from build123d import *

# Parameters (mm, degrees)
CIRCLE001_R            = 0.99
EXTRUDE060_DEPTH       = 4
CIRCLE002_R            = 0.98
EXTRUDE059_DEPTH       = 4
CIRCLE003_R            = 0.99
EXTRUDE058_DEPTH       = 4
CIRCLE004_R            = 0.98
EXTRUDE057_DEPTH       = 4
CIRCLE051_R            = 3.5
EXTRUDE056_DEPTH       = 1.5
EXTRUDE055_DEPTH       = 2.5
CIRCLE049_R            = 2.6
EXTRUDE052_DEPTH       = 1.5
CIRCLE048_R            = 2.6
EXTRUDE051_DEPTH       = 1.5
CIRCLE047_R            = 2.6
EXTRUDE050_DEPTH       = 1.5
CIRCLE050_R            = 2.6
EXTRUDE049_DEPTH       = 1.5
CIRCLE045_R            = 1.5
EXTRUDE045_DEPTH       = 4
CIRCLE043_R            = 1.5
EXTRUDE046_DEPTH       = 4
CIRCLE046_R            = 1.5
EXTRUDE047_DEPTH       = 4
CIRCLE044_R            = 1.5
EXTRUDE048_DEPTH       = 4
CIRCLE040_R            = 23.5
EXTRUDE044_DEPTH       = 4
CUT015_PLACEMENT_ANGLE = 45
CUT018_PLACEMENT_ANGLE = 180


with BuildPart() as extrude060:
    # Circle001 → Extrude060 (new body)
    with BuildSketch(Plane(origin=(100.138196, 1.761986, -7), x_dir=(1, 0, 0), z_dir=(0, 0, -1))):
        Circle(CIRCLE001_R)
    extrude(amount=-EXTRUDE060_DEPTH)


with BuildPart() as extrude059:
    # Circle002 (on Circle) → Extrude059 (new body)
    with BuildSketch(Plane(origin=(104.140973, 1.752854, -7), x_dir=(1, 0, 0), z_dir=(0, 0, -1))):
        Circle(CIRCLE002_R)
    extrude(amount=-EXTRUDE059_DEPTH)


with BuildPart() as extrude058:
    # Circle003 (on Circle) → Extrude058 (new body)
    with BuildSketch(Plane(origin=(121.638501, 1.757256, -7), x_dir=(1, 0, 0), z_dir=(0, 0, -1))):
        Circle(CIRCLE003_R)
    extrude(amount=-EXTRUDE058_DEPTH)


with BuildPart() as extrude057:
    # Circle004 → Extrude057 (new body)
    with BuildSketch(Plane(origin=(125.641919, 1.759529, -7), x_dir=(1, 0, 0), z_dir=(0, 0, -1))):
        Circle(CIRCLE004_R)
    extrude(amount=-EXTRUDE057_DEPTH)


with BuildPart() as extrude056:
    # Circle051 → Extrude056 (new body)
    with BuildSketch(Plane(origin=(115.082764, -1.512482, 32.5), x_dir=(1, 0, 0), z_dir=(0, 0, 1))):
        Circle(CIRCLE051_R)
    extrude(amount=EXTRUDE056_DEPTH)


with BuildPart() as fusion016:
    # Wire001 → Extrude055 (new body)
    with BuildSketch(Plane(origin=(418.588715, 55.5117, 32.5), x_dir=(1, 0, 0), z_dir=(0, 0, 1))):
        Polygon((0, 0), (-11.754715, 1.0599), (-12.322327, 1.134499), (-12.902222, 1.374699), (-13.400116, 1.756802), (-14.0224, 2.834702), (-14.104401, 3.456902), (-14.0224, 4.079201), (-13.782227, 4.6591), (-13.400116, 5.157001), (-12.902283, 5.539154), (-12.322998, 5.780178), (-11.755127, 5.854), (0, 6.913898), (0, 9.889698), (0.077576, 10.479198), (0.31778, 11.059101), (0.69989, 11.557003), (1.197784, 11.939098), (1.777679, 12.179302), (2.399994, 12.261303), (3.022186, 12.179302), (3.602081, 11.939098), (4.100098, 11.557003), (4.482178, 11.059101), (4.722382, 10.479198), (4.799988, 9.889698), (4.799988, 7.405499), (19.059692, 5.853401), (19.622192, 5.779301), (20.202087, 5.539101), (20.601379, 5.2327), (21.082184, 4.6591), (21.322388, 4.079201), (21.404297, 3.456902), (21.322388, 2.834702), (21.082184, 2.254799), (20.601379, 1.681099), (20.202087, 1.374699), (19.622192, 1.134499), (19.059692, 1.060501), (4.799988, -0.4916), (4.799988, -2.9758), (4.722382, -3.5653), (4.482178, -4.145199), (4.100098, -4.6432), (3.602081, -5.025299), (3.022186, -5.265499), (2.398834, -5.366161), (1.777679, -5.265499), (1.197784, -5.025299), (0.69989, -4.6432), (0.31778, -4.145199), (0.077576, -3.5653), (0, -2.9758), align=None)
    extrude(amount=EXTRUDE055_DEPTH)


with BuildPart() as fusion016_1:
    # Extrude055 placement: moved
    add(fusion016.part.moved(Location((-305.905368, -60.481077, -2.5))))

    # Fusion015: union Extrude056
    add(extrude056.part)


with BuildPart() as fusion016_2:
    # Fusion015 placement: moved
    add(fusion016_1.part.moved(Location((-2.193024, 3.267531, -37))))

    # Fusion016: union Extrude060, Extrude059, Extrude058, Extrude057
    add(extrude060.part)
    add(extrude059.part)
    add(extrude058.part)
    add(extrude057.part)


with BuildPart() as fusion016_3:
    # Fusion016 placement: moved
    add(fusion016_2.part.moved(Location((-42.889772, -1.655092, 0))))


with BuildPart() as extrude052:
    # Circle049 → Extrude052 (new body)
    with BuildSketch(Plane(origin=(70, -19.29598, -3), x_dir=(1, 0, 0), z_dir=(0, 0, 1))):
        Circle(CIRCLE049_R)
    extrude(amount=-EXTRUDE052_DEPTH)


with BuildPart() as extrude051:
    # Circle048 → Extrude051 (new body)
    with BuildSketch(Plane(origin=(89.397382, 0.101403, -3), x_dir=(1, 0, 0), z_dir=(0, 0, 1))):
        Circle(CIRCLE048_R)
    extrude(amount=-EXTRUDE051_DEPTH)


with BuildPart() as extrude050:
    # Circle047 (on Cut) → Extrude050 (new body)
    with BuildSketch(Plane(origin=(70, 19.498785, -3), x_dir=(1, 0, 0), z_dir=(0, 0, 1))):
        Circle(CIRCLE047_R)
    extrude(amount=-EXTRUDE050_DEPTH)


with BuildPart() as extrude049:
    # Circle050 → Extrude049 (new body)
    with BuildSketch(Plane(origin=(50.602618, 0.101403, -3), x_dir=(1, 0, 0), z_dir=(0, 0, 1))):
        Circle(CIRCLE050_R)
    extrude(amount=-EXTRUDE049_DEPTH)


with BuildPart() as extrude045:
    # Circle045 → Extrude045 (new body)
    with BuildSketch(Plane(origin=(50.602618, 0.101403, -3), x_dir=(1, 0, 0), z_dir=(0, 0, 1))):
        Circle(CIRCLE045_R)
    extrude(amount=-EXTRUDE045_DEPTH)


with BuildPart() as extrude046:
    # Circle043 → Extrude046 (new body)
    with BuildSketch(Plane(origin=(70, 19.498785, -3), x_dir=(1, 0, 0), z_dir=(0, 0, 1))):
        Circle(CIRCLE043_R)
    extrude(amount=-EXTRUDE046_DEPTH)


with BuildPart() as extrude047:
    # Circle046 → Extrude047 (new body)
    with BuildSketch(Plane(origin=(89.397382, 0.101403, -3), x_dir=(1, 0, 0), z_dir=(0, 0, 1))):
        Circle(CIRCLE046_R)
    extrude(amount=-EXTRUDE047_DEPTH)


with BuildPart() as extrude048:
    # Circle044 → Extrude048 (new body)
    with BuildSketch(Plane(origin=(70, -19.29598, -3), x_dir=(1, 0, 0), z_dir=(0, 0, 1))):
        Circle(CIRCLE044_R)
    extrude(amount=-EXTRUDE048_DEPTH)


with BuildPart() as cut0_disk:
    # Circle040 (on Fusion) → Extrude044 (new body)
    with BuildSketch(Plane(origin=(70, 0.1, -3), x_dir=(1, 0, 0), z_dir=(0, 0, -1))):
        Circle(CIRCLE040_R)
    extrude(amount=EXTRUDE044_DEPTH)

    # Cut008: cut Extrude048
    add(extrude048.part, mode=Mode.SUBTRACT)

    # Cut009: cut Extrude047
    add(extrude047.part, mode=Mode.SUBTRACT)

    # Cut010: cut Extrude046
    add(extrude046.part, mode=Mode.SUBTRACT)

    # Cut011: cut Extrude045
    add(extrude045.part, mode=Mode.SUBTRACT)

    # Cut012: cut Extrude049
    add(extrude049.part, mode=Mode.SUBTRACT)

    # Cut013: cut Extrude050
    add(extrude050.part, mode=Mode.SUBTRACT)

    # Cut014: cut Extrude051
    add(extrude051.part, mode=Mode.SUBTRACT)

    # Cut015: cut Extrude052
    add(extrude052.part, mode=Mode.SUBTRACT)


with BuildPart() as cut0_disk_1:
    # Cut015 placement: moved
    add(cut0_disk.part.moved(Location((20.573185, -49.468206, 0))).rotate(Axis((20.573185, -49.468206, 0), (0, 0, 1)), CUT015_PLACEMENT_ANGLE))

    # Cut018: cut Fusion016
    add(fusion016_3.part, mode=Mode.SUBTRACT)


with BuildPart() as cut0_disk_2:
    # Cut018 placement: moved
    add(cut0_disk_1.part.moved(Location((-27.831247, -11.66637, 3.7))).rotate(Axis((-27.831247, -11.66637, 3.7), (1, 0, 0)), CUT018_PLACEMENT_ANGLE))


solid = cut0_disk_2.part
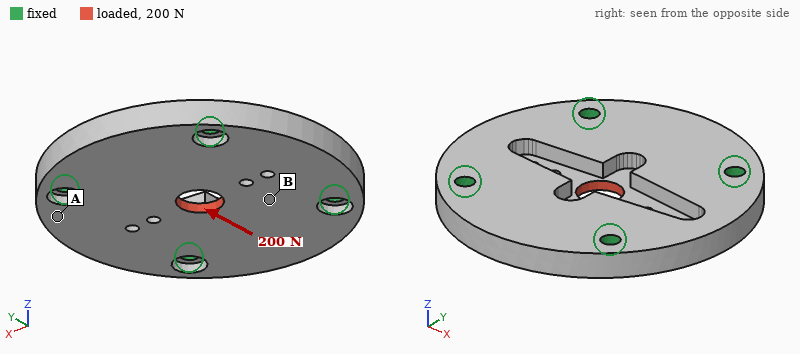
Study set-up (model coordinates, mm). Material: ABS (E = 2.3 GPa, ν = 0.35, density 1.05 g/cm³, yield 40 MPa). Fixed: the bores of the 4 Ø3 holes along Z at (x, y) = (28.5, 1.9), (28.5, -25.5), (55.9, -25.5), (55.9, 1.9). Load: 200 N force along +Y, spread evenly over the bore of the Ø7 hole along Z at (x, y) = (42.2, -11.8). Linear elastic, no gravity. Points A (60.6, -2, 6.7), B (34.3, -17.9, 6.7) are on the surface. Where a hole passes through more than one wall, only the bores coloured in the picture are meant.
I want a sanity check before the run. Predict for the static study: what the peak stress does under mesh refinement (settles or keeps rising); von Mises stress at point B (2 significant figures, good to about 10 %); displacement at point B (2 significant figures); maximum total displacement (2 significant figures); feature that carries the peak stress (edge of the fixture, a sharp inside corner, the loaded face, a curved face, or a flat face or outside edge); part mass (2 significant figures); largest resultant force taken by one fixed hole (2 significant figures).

keeps rising
2.5 MPa
13 µm
38 µm
a sharp inside corner
6.3 g
52 N
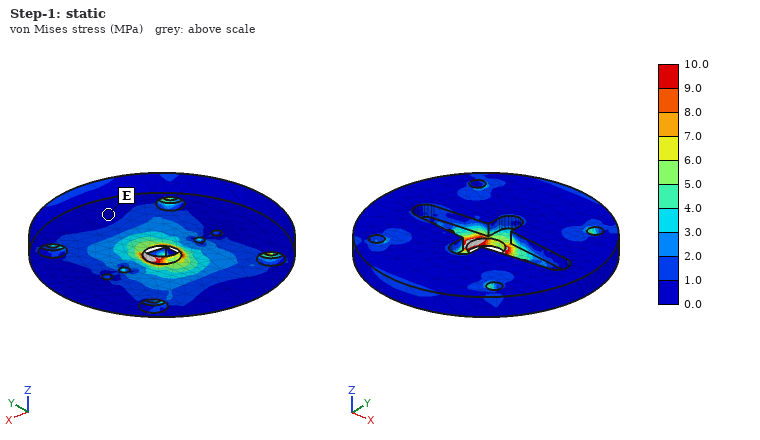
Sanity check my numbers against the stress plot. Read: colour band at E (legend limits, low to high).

0.0 to 1.0 MPa
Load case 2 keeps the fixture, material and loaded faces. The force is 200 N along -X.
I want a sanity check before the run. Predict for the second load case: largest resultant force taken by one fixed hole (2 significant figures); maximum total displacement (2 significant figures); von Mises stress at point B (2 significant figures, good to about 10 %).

53 N
31 µm
2.5 MPa
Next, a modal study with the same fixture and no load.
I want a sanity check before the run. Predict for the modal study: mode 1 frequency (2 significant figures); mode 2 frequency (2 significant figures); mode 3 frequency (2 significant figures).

4500 Hz
4900 Hz
5100 Hz
